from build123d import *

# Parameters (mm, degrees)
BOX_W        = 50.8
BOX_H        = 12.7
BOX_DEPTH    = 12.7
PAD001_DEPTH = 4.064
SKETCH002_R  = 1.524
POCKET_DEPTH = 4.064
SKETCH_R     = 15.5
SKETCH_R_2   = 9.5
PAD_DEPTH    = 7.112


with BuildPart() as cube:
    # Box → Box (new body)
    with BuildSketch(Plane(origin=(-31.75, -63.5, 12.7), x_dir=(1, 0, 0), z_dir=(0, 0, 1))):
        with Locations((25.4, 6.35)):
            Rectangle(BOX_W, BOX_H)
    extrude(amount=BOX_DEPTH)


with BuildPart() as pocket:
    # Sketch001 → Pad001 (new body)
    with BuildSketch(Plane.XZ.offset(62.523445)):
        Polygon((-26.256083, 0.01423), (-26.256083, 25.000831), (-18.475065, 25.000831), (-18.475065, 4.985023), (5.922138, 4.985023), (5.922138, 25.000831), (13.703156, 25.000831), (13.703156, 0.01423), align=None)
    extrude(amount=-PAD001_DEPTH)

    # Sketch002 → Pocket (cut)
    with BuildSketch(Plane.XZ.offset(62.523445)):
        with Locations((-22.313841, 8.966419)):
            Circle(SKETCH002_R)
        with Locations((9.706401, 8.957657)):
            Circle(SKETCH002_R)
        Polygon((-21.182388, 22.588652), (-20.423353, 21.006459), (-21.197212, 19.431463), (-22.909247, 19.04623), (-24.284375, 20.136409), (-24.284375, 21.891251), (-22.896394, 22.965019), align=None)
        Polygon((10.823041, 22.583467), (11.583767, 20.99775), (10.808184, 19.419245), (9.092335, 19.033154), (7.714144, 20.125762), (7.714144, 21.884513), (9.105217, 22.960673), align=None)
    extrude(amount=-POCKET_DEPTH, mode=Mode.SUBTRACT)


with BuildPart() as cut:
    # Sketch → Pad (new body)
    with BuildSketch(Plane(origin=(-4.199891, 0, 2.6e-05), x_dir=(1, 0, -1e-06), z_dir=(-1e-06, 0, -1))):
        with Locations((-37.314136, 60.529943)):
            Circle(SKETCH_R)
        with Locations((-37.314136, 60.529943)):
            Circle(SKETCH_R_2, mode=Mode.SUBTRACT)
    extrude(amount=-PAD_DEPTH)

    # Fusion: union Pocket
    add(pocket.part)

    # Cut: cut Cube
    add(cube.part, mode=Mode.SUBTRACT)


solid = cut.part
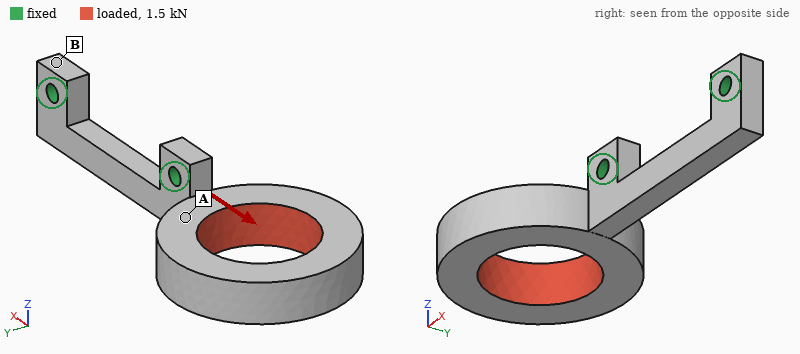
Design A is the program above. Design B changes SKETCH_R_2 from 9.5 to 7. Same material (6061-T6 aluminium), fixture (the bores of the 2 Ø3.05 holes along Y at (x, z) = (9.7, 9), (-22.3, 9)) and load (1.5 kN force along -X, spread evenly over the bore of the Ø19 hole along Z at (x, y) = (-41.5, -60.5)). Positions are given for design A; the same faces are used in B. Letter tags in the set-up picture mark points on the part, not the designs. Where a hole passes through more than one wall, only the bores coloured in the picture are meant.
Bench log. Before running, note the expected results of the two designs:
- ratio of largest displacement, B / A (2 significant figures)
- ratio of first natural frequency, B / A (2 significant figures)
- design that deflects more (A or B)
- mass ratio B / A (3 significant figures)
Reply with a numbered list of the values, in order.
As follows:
1. 0.90
2. 0.93
3. A
4. 1.20
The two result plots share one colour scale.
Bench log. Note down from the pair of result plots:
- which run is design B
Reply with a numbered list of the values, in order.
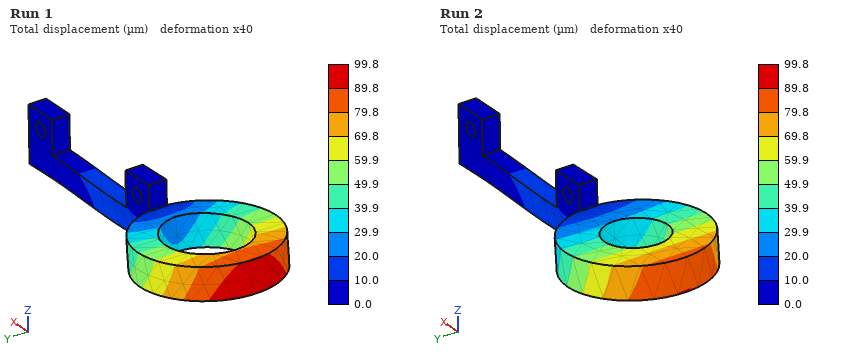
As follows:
1. Run 2
